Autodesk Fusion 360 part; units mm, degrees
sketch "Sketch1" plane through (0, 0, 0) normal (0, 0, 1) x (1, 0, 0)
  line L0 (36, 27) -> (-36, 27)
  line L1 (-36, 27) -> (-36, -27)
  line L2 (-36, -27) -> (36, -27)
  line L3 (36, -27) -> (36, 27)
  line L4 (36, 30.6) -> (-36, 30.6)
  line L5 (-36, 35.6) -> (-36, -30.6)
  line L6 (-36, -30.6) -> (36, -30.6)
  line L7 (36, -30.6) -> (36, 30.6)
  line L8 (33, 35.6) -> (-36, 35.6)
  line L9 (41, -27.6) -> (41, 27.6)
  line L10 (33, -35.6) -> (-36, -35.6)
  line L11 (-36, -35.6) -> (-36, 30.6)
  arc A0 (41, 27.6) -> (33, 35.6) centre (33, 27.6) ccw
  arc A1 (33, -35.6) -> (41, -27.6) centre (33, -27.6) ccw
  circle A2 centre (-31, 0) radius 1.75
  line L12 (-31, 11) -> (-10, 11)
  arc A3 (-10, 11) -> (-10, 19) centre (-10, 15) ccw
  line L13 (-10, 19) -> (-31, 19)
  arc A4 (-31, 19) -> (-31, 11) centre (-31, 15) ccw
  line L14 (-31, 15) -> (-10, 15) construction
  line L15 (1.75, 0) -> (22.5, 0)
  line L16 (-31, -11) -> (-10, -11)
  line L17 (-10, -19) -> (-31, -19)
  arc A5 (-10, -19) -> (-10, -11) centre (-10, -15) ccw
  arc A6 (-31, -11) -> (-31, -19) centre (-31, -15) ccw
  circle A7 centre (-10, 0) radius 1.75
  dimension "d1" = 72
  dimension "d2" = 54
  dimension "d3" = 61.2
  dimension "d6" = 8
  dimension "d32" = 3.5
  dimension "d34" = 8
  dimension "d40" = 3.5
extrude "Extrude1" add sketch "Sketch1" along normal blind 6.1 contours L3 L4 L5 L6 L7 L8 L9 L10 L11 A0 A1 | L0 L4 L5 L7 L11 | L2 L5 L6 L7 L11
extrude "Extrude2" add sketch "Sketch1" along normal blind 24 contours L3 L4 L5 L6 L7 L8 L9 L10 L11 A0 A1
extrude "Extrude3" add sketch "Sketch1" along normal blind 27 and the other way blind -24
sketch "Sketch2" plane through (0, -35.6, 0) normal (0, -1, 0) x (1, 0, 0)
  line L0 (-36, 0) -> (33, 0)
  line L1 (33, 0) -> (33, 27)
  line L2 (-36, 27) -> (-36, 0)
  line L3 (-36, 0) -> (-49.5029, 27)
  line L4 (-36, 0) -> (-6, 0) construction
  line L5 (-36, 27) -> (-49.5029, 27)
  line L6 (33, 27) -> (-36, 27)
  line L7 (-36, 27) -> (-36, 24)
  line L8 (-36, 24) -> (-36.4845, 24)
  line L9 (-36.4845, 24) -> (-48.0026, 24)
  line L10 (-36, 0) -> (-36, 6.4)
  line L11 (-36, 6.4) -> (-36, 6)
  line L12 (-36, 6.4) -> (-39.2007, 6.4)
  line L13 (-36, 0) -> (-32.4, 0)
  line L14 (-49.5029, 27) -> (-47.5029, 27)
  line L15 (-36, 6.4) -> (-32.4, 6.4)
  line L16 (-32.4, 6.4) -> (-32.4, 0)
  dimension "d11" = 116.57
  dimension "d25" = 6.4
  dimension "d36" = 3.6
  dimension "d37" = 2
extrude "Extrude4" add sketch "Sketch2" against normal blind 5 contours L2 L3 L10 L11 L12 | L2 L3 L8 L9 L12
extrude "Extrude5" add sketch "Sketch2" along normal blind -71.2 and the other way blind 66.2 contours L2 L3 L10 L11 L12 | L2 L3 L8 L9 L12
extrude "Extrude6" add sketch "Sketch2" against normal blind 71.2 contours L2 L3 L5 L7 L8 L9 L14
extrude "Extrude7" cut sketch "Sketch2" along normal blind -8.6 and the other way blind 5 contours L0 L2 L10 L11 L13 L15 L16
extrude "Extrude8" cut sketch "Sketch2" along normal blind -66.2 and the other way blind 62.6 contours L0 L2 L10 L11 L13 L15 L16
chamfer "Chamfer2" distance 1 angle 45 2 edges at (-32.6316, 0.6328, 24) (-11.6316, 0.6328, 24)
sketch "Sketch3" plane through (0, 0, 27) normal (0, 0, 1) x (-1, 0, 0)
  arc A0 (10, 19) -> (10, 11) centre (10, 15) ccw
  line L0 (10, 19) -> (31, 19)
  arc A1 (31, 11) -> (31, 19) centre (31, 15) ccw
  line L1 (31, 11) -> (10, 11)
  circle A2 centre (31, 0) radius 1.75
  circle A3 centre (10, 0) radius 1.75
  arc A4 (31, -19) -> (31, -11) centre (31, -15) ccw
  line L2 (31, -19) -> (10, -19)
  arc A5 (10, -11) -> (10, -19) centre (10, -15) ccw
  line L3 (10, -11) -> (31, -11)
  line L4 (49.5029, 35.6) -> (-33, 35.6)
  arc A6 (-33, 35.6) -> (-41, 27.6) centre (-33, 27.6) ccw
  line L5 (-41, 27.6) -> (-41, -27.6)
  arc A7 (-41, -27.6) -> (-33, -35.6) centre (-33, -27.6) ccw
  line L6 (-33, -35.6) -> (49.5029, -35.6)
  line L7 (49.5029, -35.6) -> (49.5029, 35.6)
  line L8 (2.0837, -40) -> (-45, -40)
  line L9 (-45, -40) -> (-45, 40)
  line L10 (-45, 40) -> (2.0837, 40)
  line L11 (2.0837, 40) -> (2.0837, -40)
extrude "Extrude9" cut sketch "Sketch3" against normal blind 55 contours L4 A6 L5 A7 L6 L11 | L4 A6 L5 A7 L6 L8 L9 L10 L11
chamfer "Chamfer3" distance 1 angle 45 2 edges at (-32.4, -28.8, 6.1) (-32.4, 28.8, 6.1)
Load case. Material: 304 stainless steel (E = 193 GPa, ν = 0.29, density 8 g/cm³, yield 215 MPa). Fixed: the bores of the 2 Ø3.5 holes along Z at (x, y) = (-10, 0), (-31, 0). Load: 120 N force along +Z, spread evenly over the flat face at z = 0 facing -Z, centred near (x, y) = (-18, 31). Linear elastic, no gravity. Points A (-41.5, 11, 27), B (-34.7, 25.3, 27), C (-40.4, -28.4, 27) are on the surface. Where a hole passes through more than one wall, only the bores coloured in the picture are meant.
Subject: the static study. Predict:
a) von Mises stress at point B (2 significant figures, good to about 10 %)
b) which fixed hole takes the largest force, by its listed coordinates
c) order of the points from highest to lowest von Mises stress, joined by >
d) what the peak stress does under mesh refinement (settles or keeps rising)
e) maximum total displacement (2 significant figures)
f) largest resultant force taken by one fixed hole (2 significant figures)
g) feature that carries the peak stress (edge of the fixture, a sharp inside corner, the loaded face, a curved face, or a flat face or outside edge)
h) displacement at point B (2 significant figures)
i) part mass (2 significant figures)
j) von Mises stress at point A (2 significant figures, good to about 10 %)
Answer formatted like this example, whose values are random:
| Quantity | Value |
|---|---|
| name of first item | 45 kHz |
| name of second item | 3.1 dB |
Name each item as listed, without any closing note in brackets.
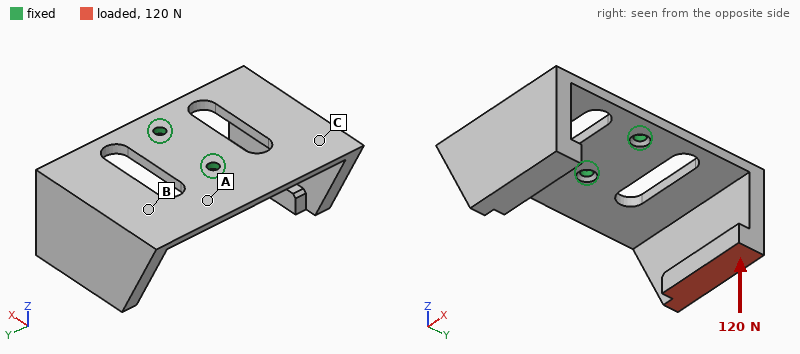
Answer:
| Quantity | Value |
|---|---|
| von Mises stress at point B | 21 MPa |
| which fixed hole takes the largest force, by its listed coordinates | (-10, 0) |
| order of the points from highest to lowest von Mises stress, joined by > | A > B > C |
| what the peak stress does under mesh refinement | keeps rising |
| maximum total displacement | 0.23 mm |
| largest resultant force taken by one fixed hole | 71 N |
| feature that carries the peak stress | edge of the fixture |
| displacement at point B | 0.090 mm |
| part mass | 160 g |
| von Mises stress at point A | 63 MPa |
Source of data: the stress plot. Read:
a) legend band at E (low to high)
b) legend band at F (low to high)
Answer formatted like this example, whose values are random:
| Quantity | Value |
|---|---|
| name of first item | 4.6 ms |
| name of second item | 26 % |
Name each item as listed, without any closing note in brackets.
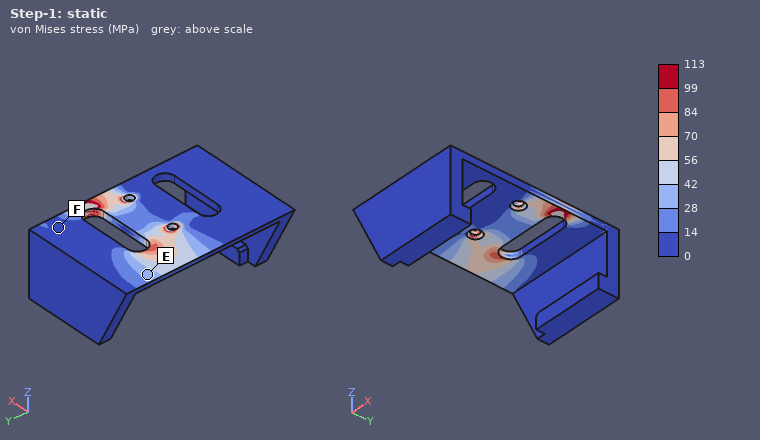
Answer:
| Quantity | Value |
|---|---|
| legend band at E | 28 to 42 MPa |
| legend band at F | 0 to 14 MPa |
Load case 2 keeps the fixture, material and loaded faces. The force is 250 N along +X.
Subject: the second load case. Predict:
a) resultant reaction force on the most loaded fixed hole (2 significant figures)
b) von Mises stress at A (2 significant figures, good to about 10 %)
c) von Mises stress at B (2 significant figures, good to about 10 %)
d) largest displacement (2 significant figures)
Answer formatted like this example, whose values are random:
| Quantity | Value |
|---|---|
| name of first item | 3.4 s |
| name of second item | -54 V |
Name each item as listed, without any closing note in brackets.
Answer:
| Quantity | Value |
|---|---|
| resultant reaction force on the most loaded fixed hole | 430 N |
| von Mises stress at A | 42 MPa |
| von Mises stress at B | 48 MPa |
| largest displacement | 0.16 mm |
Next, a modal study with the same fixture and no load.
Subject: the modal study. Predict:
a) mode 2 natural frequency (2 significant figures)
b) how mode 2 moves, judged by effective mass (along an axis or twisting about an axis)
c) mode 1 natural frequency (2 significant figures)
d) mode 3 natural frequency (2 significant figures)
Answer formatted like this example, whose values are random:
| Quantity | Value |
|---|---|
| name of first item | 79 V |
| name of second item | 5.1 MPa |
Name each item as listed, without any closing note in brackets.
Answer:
| Quantity | Value |
|---|---|
| mode 2 natural frequency | 550 Hz |
| how mode 2 moves, judged by effective mass | along Z |
| mode 1 natural frequency | 480 Hz |
| mode 3 natural frequency | 1300 Hz |
